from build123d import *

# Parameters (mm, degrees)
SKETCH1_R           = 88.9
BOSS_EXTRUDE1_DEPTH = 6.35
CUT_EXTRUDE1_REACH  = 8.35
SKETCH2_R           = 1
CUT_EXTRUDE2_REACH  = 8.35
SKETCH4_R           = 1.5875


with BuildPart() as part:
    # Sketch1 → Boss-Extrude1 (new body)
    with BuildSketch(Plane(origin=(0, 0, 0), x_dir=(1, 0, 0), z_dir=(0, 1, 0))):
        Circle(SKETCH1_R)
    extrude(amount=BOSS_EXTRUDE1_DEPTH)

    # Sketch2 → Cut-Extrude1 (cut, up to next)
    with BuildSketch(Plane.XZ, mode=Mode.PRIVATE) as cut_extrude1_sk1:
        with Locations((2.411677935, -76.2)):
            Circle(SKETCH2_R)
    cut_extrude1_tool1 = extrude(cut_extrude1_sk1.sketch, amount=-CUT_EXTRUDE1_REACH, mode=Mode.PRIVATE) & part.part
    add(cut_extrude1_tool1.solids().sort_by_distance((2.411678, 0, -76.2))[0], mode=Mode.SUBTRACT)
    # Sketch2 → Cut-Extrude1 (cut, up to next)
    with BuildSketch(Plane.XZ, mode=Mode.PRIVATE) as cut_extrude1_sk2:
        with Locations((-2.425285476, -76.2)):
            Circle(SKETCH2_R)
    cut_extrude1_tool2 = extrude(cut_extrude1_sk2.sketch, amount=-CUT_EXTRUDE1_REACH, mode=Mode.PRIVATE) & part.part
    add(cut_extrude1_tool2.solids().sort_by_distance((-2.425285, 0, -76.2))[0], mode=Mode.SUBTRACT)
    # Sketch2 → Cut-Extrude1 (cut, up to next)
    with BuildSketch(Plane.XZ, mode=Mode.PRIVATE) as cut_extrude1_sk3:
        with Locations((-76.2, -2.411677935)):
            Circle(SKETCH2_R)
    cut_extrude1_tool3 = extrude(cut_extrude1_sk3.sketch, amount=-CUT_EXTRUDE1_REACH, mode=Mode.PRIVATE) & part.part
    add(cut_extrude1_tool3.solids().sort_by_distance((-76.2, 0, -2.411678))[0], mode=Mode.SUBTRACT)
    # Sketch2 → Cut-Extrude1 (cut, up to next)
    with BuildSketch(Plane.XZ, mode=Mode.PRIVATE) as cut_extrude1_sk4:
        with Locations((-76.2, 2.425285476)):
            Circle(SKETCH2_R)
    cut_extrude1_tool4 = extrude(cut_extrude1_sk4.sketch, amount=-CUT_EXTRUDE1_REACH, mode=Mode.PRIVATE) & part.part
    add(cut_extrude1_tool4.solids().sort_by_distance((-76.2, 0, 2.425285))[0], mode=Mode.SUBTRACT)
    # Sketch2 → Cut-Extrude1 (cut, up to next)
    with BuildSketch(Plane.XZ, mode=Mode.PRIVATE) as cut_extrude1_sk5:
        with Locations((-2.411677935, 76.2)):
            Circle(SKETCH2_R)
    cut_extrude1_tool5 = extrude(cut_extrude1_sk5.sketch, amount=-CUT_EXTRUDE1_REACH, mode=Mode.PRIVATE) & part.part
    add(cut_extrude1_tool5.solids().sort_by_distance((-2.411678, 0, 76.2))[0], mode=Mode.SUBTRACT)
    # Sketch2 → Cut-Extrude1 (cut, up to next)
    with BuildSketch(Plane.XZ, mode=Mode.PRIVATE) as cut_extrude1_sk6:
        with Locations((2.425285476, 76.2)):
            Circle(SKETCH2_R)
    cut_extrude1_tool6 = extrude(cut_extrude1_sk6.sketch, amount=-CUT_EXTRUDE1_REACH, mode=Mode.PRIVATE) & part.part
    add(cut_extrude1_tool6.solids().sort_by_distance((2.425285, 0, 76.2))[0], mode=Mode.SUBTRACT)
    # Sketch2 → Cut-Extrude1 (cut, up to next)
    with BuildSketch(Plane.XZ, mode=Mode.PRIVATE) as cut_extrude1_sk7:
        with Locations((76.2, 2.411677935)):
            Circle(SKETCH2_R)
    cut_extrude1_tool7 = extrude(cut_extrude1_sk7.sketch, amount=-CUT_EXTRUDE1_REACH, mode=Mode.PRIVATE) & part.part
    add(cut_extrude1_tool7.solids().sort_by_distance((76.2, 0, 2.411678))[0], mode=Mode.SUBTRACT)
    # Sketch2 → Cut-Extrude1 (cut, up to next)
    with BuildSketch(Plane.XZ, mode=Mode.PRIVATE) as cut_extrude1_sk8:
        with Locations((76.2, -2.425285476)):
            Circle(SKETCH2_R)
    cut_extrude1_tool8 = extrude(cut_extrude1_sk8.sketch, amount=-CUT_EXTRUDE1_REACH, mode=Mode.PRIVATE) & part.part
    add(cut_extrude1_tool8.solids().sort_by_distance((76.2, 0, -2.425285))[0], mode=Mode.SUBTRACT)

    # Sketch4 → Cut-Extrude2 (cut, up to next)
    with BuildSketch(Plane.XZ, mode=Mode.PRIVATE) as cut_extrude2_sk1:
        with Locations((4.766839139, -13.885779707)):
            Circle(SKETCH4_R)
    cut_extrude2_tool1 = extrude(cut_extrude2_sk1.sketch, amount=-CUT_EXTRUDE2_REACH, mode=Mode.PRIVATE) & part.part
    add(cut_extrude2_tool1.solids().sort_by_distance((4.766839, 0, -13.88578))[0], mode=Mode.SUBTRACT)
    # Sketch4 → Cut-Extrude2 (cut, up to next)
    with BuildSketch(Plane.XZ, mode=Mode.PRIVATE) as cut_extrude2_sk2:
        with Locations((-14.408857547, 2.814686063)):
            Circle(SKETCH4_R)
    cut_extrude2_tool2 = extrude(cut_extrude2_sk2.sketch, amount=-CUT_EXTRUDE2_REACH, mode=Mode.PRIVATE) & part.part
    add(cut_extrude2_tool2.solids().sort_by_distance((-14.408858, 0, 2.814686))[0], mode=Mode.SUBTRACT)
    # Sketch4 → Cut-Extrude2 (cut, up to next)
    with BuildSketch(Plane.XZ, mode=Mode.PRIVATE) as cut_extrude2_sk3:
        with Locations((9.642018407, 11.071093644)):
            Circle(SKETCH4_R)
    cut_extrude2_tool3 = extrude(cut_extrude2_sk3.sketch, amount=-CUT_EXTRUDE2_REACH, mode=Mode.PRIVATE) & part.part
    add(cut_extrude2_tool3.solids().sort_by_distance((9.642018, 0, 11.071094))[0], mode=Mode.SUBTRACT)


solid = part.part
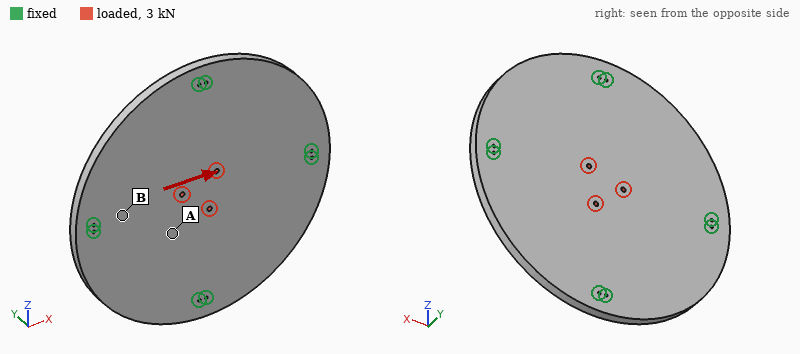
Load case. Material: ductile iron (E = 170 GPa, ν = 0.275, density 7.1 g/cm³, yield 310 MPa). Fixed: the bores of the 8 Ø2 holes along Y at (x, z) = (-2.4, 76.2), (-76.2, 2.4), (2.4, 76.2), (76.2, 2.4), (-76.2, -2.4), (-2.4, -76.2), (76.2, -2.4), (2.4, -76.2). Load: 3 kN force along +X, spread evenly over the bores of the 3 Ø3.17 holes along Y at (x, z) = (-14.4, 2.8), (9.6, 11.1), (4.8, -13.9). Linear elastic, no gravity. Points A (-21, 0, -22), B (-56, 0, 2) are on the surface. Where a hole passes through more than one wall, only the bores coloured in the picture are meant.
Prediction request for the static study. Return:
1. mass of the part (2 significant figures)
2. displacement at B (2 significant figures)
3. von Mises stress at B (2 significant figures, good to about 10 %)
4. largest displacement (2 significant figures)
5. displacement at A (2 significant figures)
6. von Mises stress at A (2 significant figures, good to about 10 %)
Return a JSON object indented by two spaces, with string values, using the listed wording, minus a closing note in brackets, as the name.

{
  "mass of the part": "1.1 kg",
  "displacement at B": "0.76 µm",
  "von Mises stress at B": "5.2 MPa",
  "largest displacement": "2.3 µm",
  "displacement at A": "1.3 µm",
  "von Mises stress at A": "2.6 MPa"
}
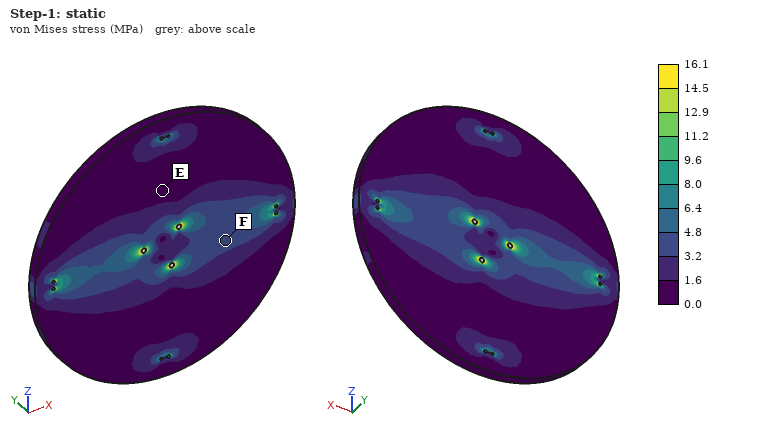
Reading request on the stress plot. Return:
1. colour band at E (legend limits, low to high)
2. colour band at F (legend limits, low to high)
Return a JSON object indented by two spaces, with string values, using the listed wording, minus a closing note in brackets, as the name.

{
  "colour band at E": "0.0 to 1.6 MPa",
  "colour band at F": "3.2 to 4.8 MPa"
}
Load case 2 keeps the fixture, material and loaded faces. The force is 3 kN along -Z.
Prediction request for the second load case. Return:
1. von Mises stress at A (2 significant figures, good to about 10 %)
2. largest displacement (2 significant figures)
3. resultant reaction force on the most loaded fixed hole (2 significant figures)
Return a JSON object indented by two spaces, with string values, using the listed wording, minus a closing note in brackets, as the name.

{
  "von Mises stress at A": "2.8 MPa",
  "largest displacement": "2.3 µm",
  "resultant reaction force on the most loaded fixed hole": "480 N"
}
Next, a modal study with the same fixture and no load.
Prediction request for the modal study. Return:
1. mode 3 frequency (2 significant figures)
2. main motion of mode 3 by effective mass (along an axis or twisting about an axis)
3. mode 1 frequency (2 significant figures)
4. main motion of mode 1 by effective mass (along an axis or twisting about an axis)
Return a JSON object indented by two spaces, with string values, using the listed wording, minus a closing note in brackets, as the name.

{
  "mode 3 frequency": "2100 Hz",
  "main motion of mode 3 by effective mass": "twisting about X",
  "mode 1 frequency": "1700 Hz",
  "main motion of mode 1 by effective mass": "along Y"
}
